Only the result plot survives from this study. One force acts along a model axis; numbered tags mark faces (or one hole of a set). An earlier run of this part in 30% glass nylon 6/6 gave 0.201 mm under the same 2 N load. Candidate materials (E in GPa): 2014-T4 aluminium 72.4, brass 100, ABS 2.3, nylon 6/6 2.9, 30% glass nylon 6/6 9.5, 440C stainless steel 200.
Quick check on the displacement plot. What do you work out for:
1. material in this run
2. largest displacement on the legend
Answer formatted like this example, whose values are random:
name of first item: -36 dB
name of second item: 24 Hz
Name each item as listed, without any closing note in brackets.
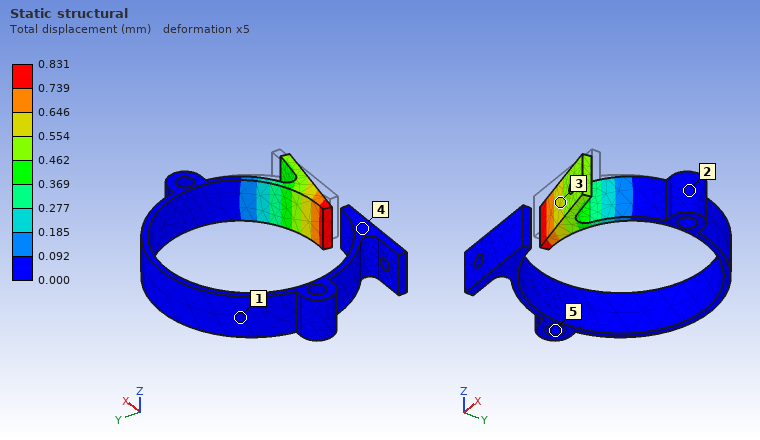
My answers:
material in this run: ABS
largest displacement on the legend: 0.831 mm
